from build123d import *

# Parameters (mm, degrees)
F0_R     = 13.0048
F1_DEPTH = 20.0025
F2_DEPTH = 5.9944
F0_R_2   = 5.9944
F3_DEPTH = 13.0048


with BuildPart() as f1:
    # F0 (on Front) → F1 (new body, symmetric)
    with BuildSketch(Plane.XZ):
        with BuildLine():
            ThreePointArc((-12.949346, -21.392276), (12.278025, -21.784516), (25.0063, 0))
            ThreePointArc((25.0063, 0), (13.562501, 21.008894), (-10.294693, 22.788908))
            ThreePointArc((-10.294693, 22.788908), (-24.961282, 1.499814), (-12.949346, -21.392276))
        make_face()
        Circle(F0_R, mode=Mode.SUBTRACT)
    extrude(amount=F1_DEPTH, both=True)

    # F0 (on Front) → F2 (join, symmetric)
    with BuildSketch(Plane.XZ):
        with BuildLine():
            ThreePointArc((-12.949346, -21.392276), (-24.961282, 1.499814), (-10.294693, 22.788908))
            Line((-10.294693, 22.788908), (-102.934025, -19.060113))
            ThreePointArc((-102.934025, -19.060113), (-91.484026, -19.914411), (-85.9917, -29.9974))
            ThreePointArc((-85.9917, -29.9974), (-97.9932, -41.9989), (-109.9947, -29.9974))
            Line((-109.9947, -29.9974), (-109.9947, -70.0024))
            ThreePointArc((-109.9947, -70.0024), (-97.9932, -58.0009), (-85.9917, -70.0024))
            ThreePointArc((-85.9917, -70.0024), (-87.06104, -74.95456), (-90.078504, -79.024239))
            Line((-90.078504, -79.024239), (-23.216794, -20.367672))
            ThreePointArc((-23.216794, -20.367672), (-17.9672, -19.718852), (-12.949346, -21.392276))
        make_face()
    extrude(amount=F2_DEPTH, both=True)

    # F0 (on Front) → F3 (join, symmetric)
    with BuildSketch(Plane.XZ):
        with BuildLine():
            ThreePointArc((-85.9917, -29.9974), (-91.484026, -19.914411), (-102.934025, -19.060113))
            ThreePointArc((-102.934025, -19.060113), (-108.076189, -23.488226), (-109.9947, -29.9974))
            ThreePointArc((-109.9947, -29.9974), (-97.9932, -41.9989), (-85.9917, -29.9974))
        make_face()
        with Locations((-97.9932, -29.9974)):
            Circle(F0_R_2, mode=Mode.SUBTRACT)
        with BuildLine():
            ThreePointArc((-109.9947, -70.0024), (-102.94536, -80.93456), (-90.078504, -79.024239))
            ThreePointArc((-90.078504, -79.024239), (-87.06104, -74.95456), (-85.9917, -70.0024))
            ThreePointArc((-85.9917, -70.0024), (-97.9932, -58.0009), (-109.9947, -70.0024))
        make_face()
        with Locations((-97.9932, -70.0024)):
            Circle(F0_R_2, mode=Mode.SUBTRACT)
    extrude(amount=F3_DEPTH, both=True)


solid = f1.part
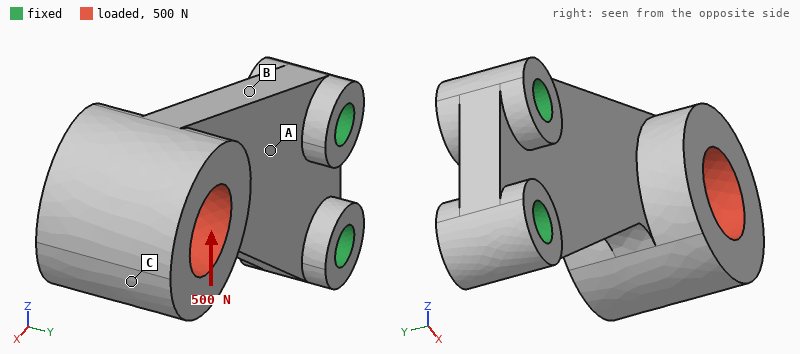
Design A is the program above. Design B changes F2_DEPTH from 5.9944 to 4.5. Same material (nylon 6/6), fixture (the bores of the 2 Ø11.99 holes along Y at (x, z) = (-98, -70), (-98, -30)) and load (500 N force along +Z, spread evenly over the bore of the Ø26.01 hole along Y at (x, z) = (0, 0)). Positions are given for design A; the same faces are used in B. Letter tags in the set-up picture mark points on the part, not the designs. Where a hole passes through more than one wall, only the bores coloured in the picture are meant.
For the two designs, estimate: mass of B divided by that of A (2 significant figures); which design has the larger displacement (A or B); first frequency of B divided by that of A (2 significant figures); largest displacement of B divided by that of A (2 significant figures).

0.91
B
0.67
1.3
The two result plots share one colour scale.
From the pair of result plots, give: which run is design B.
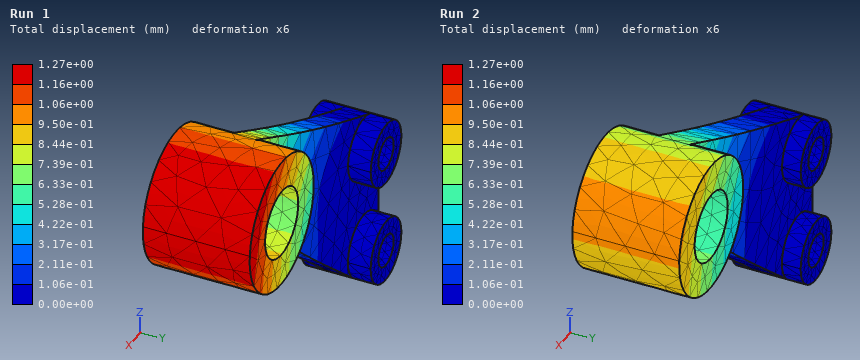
Run 1
